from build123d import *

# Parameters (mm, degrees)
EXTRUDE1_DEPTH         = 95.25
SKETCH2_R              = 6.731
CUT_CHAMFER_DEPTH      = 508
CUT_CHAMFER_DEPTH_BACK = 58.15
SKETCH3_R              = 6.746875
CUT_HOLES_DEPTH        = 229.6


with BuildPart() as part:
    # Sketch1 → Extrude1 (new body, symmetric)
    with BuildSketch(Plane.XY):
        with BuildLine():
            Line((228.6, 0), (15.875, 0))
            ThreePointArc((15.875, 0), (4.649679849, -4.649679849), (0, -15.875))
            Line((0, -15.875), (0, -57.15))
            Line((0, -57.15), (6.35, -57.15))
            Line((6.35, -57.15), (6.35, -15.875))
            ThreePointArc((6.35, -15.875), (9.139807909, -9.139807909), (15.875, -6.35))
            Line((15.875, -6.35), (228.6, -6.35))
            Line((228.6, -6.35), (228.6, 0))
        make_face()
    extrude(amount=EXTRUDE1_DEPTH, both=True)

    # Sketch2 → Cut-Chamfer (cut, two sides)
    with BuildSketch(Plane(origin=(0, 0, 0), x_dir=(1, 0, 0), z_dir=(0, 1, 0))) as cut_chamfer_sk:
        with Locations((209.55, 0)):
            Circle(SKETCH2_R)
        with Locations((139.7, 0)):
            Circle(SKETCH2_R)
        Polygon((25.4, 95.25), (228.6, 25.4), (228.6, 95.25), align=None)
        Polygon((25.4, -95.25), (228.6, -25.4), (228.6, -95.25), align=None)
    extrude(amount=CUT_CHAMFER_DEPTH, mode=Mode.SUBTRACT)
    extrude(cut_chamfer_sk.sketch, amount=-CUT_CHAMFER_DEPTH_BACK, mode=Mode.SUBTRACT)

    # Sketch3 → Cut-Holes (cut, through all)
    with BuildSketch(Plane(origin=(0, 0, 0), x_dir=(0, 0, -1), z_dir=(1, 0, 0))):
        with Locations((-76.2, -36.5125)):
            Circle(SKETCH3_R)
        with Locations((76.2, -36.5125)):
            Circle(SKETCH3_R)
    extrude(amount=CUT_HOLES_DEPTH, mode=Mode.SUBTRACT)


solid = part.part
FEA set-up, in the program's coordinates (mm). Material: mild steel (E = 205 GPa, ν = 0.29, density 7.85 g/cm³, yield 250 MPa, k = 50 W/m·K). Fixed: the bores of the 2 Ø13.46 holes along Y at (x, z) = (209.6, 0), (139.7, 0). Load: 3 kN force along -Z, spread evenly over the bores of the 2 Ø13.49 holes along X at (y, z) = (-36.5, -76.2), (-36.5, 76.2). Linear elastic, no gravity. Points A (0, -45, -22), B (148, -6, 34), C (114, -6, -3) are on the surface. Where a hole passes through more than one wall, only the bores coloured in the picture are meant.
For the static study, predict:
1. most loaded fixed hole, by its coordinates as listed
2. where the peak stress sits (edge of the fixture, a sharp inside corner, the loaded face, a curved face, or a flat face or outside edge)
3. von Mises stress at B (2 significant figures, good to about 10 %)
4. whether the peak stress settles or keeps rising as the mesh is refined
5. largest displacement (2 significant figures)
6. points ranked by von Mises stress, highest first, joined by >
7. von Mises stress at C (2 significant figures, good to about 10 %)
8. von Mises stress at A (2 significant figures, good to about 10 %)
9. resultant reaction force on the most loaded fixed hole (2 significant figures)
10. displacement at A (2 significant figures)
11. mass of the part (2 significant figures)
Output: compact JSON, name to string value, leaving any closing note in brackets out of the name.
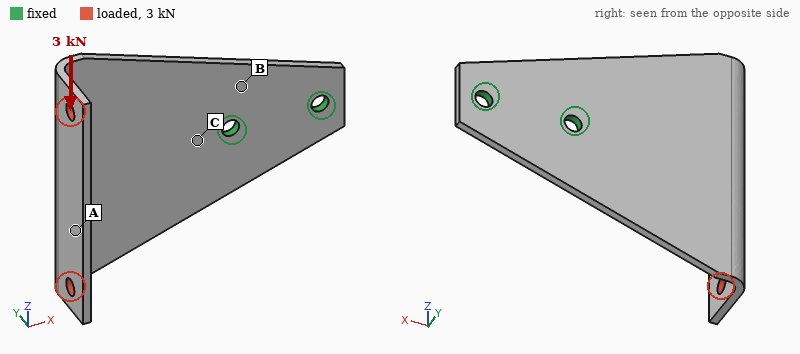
{"most loaded fixed hole, by its coordinates as listed": "(139.7, 0)", "where the peak stress sits": "edge of the fixture", "von Mises stress at B": "68 MPa", "whether the peak stress settles or keeps rising as the mesh is refined": "keeps rising", "largest displacement": "1.5 mm", "points ranked by von Mises stress, highest first, joined by >": "C > B > A", "von Mises stress at C": "130 MPa", "von Mises stress at A": "30 MPa", "resultant reaction force on the most loaded fixed hole": "7.8 kN", "displacement at A": "0.67 mm", "mass of the part": "1.9 kg"}
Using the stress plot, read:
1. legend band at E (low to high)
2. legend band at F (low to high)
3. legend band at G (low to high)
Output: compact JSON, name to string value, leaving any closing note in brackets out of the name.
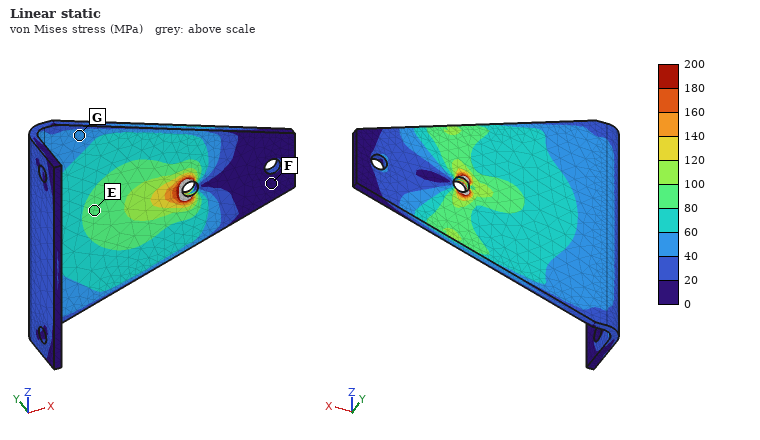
{"legend band at E": "80 to 100 MPa", "legend band at F": "0 to 20 MPa", "legend band at G": "40 to 60 MPa"}
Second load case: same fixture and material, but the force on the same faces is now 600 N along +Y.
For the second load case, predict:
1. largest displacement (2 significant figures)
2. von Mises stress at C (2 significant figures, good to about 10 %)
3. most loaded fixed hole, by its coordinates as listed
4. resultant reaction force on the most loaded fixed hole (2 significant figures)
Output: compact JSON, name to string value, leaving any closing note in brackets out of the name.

{"largest displacement": "1.1 mm", "von Mises stress at C": "81 MPa", "most loaded fixed hole, by its coordinates as listed": "(139.7, 0)", "resultant reaction force on the most loaded fixed hole": "980 N"}
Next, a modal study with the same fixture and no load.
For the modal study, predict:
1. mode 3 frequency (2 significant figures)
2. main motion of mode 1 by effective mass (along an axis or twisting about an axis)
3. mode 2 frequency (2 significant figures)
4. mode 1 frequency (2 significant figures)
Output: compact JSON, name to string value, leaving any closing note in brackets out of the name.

{"mode 3 frequency": "760 Hz", "main motion of mode 1 by effective mass": "along Y", "mode 2 frequency": "240 Hz", "mode 1 frequency": "140 Hz"}
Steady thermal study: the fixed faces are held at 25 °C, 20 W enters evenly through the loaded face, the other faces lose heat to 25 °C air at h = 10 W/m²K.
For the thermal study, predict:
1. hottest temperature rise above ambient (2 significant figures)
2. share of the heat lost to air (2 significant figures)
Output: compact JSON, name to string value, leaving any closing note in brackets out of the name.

{"hottest temperature rise above ambient": "47 K", "share of the heat lost to air": "69 %"}
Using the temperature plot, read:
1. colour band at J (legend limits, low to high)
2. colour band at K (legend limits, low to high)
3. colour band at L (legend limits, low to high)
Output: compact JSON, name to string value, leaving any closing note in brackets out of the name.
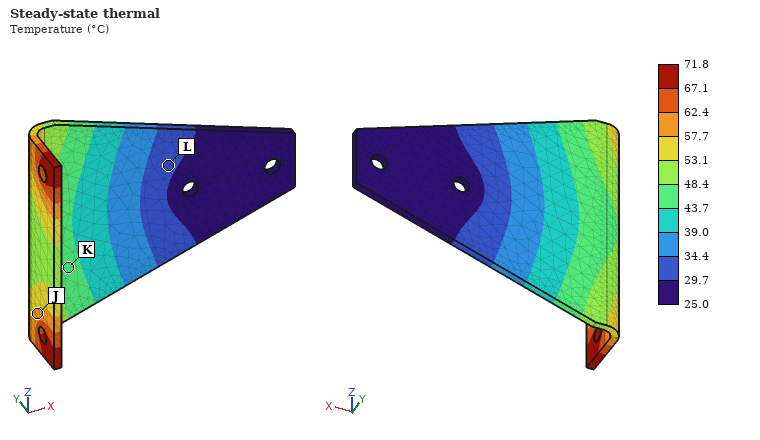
{"colour band at J": "57.7 to 62.4 °C", "colour band at K": "43.7 to 48.4 °C", "colour band at L": "29.7 to 34.4 °C"}
